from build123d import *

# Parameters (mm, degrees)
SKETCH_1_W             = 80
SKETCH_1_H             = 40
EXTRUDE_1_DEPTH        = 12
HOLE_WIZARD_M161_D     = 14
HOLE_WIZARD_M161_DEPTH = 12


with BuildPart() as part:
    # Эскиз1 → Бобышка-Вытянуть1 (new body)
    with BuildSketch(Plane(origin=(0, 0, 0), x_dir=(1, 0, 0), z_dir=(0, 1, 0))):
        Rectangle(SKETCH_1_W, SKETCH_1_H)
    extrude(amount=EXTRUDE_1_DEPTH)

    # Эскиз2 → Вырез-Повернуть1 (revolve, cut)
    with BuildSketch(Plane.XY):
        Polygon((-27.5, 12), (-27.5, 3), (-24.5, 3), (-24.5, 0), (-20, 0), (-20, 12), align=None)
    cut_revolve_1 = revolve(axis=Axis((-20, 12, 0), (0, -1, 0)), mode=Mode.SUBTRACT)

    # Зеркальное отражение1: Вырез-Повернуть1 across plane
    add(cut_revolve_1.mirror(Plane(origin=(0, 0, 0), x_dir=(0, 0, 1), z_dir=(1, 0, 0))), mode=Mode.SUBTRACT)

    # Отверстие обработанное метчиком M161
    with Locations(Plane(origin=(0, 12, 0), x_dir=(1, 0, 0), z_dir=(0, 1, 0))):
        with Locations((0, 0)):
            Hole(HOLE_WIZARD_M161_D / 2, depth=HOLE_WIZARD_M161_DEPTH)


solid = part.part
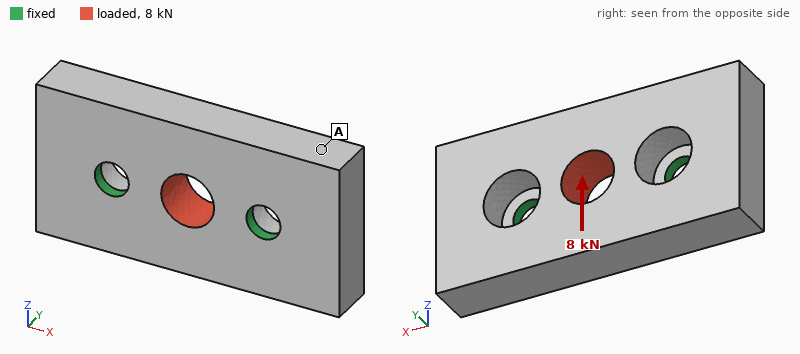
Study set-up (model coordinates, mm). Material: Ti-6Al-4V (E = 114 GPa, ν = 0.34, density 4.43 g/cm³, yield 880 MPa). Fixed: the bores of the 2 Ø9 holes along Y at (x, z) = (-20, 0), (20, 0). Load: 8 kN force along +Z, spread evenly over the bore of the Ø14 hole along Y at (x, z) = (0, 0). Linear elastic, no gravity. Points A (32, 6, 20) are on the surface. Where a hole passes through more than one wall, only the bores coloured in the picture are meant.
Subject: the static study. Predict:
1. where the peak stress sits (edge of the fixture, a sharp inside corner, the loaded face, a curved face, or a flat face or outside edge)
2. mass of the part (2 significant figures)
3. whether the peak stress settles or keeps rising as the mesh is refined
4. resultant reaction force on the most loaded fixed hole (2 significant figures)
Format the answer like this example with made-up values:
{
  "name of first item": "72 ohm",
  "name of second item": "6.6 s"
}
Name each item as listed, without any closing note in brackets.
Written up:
{
  "where the peak stress sits": "edge of the fixture",
  "mass of the part": "150 g",
  "whether the peak stress settles or keeps rising as the mesh is refined": "keeps rising",
  "resultant reaction force on the most loaded fixed hole": "4.0 kN"
}
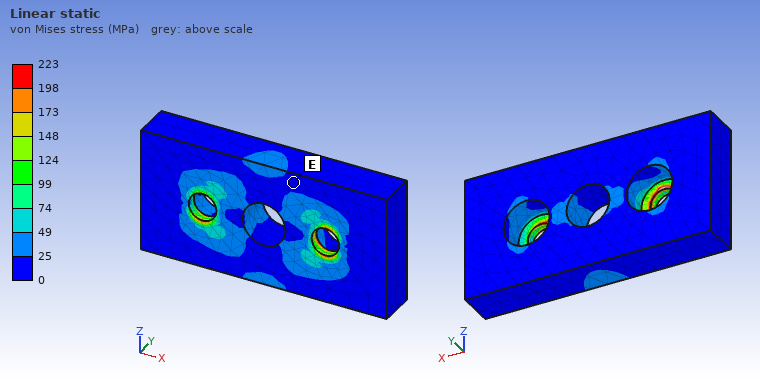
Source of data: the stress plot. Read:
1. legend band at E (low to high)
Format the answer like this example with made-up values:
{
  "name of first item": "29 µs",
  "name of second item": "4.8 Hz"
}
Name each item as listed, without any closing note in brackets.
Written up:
{
  "legend band at E": "0 to 25 MPa"
}
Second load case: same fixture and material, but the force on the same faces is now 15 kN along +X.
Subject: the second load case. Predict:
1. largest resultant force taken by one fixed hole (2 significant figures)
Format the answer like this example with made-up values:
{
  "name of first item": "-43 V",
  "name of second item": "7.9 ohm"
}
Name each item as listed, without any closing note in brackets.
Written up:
{
  "largest resultant force taken by one fixed hole": "7.7 kN"
}
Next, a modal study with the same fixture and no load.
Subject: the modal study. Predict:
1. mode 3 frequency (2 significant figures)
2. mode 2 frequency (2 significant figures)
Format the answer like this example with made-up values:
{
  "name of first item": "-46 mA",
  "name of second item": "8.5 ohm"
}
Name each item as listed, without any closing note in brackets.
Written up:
{
  "mode 3 frequency": "9700 Hz",
  "mode 2 frequency": "9100 Hz"
}
